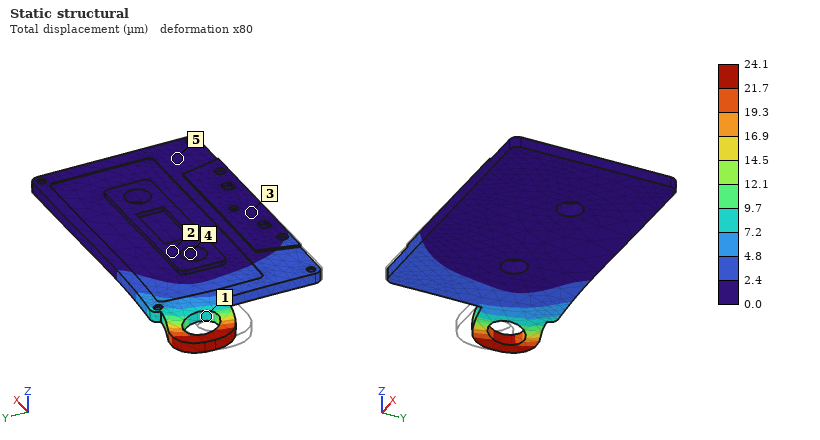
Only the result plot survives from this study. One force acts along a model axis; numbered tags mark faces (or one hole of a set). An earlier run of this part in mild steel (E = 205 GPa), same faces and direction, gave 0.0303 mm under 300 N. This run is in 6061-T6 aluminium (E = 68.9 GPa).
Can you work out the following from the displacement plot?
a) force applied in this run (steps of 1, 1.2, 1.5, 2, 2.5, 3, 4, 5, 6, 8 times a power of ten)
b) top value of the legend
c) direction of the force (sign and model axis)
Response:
80 N
24.1 µm
+Y
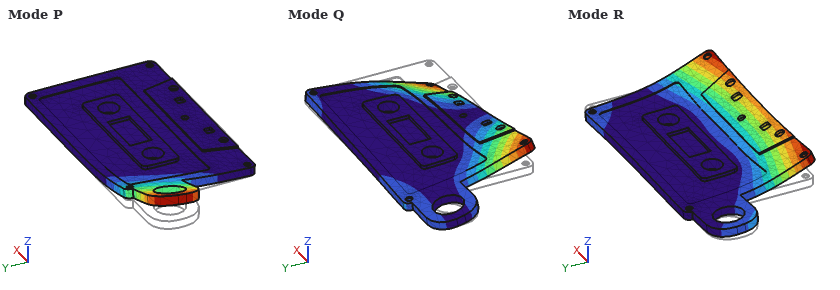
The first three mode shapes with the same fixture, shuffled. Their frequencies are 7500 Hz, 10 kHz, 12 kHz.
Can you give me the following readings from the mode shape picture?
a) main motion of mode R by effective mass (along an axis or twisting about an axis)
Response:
along Z
